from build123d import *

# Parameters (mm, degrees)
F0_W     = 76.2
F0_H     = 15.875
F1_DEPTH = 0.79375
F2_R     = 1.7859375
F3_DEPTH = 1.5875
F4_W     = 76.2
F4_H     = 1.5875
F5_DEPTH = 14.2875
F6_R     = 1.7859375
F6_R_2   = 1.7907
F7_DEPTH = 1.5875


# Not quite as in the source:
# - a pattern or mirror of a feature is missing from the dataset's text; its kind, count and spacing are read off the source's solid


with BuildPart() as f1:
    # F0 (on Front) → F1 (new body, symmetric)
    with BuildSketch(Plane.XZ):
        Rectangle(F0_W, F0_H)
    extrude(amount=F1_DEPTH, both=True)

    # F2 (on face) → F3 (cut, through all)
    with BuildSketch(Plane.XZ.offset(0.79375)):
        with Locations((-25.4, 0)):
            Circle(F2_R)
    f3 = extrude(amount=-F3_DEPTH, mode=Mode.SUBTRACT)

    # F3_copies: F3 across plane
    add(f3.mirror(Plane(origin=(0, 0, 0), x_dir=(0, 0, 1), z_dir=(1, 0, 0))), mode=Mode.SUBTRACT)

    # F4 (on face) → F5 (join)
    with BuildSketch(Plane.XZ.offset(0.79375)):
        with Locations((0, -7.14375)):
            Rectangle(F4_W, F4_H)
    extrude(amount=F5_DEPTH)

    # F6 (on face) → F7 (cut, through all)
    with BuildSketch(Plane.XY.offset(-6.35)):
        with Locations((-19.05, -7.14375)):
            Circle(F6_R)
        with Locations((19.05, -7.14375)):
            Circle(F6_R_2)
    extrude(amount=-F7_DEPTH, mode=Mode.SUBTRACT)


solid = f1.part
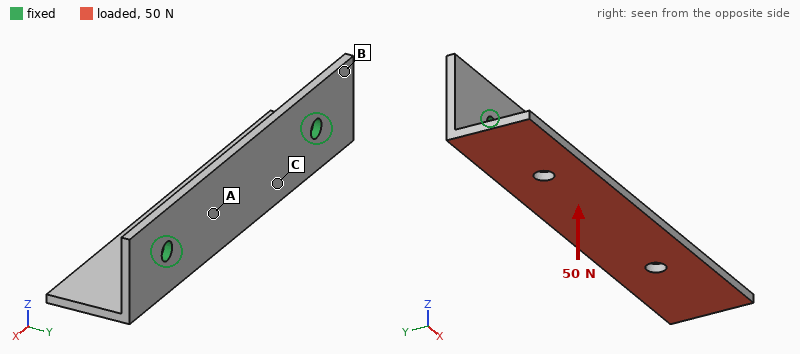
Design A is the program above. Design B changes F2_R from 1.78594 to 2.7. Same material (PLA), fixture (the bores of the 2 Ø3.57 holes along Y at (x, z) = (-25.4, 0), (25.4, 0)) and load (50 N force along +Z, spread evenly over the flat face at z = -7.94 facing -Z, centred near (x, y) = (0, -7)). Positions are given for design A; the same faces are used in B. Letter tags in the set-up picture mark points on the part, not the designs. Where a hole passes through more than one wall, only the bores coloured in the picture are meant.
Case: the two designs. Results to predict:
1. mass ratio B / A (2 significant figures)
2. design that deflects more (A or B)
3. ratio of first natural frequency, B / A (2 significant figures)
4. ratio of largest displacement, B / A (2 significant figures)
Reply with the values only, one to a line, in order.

0.99
A
1.1
0.85
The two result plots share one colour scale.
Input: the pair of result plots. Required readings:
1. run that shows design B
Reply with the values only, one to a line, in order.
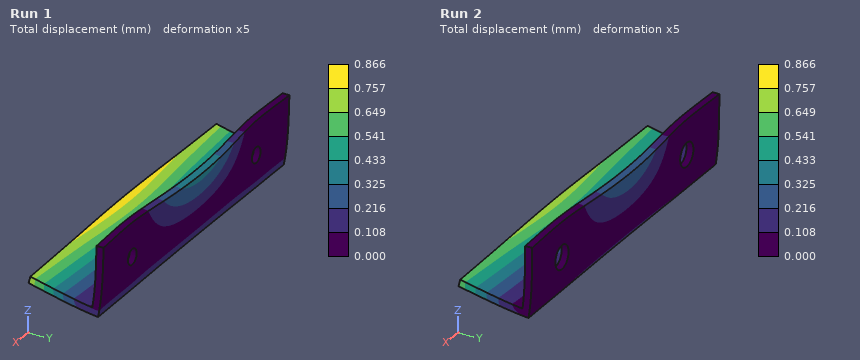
Run 2
